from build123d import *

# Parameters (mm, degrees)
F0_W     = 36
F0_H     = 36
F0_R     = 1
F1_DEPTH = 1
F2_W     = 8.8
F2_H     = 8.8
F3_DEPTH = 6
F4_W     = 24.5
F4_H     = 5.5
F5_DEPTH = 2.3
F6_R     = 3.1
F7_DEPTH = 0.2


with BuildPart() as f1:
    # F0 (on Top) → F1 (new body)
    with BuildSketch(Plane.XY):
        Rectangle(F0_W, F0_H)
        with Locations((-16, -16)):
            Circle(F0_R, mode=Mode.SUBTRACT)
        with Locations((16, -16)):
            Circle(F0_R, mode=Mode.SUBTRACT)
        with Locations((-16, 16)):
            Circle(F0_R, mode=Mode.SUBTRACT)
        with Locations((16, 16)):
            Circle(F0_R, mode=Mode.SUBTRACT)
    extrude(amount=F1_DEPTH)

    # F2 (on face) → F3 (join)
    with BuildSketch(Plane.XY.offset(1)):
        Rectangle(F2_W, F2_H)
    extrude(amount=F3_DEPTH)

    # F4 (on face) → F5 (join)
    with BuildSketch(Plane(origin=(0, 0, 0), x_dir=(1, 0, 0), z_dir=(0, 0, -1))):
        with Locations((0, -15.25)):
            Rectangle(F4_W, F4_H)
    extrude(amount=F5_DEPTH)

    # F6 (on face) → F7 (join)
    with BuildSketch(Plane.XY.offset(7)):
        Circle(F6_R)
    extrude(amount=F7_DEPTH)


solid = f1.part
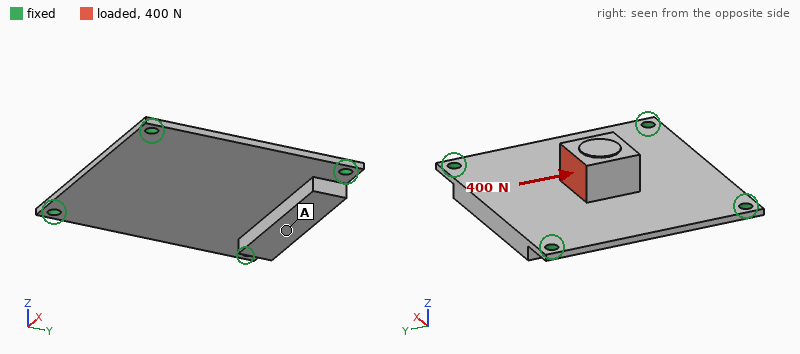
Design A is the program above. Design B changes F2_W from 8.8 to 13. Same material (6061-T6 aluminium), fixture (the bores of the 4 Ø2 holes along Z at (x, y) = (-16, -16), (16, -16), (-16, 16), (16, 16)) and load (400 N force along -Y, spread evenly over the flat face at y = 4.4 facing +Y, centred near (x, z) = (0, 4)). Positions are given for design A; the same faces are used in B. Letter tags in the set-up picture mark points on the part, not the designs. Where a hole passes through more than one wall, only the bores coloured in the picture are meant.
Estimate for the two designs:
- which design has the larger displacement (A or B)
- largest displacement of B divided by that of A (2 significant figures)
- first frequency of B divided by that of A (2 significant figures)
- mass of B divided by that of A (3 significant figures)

A
0.81
0.96
1.11
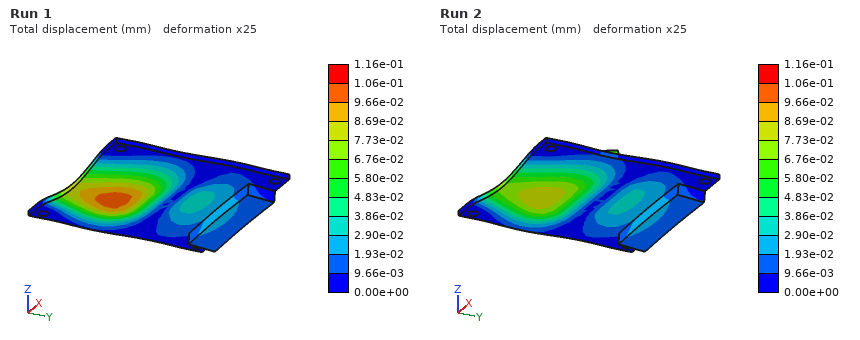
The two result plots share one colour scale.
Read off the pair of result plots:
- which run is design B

Run 2
